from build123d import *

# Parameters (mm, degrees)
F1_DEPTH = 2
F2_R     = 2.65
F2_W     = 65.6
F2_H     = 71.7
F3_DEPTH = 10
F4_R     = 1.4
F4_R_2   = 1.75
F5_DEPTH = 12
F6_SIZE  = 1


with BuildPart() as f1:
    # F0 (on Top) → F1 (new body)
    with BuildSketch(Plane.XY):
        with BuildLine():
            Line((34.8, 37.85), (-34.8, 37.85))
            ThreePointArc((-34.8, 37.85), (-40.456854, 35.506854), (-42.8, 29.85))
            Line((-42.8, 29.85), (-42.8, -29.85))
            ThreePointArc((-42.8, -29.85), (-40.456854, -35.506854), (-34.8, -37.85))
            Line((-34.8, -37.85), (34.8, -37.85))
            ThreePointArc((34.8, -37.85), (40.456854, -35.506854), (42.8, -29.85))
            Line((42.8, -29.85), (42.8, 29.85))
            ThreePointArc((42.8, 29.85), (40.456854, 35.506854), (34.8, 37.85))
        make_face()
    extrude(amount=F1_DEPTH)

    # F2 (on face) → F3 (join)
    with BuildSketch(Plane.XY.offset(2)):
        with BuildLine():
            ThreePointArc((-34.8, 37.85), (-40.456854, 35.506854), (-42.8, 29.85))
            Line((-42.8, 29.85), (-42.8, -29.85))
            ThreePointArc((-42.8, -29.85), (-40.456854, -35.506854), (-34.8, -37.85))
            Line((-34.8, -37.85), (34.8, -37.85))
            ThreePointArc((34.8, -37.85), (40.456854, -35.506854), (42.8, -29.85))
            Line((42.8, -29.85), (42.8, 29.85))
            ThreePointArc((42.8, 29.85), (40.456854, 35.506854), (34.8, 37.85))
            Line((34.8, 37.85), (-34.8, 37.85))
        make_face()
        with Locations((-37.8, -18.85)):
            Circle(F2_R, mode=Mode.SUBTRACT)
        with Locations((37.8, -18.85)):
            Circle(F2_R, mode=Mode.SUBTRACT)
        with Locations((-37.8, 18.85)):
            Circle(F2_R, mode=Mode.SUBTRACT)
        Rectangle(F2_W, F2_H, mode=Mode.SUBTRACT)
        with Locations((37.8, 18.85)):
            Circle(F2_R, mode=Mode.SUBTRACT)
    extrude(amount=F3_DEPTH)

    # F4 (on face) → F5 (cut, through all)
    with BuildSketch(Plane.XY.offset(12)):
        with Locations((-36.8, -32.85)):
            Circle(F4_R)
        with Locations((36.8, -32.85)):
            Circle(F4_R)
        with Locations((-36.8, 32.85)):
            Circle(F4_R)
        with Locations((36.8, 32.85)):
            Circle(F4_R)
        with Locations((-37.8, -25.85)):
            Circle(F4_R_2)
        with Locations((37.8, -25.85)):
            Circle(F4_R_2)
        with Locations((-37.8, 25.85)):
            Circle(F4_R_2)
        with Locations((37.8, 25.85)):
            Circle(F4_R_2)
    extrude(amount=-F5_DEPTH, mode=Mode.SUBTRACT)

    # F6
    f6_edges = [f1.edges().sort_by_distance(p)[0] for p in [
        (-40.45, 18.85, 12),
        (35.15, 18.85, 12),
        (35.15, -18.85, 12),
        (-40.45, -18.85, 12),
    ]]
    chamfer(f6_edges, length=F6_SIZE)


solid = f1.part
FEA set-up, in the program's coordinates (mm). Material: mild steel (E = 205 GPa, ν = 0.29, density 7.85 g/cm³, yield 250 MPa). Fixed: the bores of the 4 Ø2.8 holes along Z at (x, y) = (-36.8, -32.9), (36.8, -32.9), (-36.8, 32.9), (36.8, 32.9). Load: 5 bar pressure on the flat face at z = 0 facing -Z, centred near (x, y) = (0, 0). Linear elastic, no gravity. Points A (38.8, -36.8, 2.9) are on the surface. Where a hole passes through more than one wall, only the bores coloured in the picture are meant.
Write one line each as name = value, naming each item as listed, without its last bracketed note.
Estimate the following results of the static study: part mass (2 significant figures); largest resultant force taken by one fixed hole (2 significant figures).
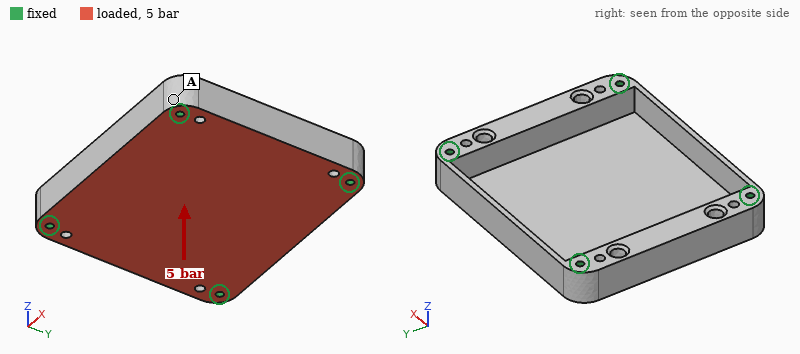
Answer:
part mass = 220 g
largest resultant force taken by one fixed hole = 880 N
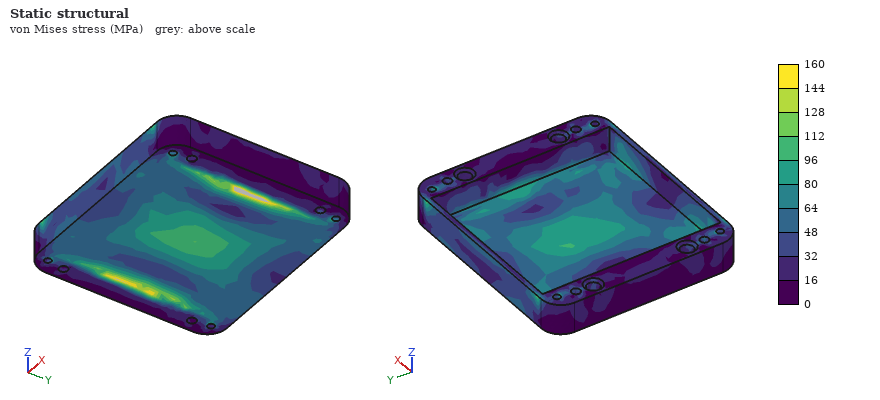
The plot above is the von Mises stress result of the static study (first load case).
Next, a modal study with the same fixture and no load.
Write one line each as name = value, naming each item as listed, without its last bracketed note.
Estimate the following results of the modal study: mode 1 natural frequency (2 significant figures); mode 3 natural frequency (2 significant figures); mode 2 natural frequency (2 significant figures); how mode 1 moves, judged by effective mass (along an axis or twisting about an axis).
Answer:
mode 1 natural frequency = 2900 Hz
mode 3 natural frequency = 6700 Hz
mode 2 natural frequency = 5000 Hz
how mode 1 moves, judged by effective mass = along Z
